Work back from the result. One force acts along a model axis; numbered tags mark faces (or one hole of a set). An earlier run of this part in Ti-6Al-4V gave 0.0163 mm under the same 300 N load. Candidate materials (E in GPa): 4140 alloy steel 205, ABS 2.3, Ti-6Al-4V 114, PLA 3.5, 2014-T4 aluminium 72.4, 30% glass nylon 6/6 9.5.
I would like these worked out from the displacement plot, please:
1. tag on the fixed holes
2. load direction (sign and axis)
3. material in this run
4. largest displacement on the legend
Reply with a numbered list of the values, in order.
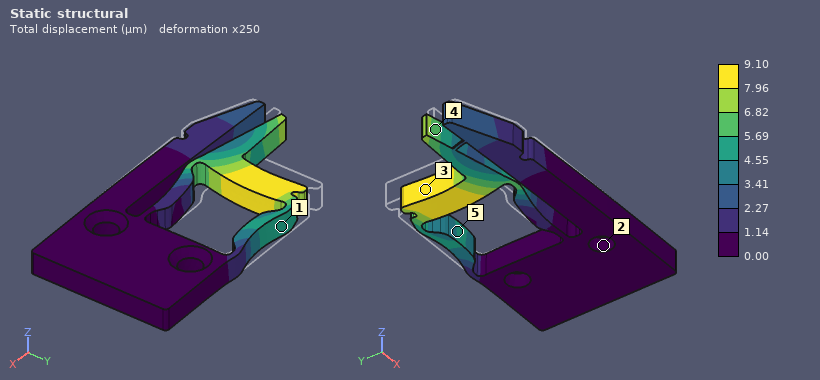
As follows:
1. 2
2. +X
3. 4140 alloy steel
4. 9.10 µm
